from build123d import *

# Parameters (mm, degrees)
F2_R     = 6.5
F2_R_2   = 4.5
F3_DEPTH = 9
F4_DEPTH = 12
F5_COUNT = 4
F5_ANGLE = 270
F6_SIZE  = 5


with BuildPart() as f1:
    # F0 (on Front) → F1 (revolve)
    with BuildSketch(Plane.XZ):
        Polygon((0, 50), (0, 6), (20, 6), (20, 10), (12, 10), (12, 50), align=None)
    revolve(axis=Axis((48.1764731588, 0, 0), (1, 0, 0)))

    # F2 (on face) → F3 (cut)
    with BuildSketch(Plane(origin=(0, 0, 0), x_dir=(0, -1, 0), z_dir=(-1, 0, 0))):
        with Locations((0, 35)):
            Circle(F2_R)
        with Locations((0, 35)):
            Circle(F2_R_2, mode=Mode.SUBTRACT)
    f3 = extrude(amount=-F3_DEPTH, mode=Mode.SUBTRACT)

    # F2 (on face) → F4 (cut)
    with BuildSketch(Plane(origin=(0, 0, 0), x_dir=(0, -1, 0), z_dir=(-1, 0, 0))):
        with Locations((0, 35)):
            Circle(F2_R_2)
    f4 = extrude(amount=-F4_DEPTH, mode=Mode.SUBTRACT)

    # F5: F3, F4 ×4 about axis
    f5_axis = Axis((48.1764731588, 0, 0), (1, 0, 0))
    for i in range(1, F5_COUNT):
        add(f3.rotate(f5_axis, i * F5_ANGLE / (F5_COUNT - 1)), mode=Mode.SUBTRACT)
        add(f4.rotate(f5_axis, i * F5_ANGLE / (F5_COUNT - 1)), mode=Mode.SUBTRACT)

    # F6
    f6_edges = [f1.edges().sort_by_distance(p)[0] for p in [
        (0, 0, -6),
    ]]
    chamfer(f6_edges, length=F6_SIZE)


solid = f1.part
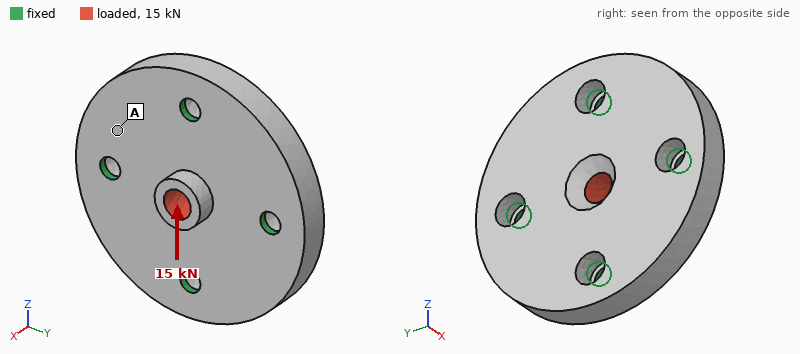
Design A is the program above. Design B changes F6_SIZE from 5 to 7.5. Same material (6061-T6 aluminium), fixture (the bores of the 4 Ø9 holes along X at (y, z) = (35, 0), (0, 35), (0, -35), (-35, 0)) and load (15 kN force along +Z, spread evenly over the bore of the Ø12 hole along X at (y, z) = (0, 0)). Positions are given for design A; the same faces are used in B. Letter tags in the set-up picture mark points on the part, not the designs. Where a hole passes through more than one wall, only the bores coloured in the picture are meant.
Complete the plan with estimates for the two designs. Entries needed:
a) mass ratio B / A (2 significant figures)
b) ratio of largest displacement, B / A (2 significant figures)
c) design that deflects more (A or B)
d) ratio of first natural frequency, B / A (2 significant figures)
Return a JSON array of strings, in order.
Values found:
["0.99", "1.2", "B", "0.98"]
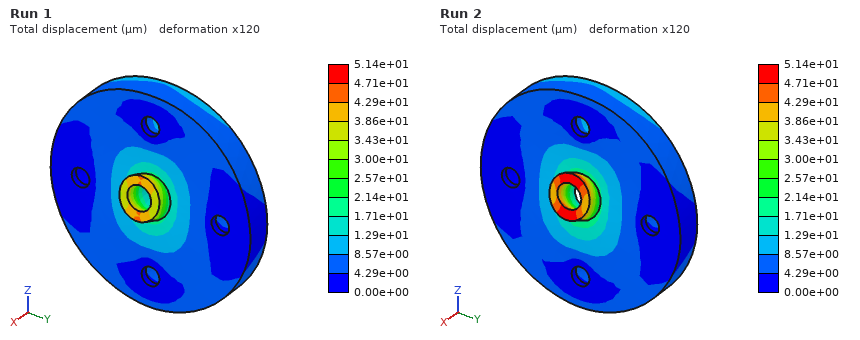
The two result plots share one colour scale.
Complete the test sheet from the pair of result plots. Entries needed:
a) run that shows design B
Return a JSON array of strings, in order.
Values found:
["Run 2"]
